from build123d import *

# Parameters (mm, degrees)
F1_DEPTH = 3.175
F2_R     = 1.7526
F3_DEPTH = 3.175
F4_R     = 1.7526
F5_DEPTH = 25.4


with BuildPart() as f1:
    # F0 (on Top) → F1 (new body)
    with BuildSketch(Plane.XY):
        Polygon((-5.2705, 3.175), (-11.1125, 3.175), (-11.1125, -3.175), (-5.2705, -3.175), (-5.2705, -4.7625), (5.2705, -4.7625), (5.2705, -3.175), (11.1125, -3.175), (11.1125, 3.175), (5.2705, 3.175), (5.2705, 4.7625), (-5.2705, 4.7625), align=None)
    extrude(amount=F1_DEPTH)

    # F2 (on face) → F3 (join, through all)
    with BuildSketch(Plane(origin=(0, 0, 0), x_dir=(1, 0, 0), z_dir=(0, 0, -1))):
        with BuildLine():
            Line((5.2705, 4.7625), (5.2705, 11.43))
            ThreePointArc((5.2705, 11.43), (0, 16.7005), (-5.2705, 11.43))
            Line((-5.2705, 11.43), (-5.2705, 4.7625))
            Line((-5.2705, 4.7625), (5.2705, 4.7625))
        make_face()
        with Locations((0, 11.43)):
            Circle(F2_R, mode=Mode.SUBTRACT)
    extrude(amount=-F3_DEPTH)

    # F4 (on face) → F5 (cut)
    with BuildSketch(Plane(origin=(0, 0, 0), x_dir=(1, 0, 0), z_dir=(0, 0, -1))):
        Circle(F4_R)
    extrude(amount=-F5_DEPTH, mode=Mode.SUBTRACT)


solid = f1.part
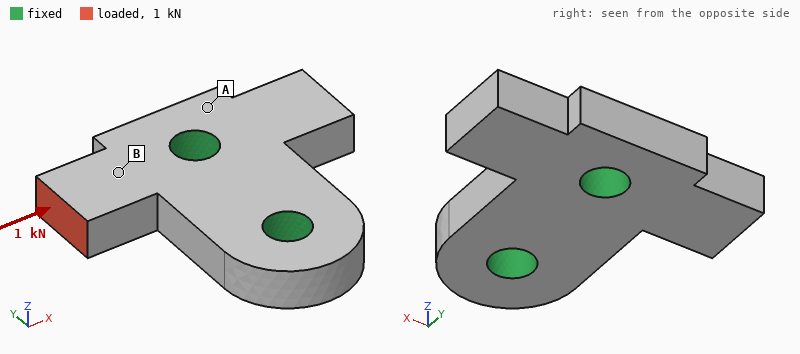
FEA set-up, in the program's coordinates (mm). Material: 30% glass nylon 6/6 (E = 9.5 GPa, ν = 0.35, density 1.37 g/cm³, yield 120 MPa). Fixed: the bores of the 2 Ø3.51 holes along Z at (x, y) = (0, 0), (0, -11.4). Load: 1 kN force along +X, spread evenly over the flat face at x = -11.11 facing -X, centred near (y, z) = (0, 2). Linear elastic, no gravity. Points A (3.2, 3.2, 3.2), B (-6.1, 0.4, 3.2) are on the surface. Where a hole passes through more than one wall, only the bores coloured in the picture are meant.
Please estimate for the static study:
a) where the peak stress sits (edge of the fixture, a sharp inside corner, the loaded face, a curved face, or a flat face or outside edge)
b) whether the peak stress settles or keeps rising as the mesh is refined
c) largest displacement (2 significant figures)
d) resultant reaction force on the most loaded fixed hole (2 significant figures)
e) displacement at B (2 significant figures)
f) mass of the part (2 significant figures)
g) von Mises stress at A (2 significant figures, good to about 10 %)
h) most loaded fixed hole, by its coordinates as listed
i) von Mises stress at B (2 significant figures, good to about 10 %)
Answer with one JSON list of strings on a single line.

["edge of the fixture", "keeps rising", "56 µm", "960 N", "26 µm", "1.2 g", "7.7 MPa", "(0, 0)", "46 MPa"]
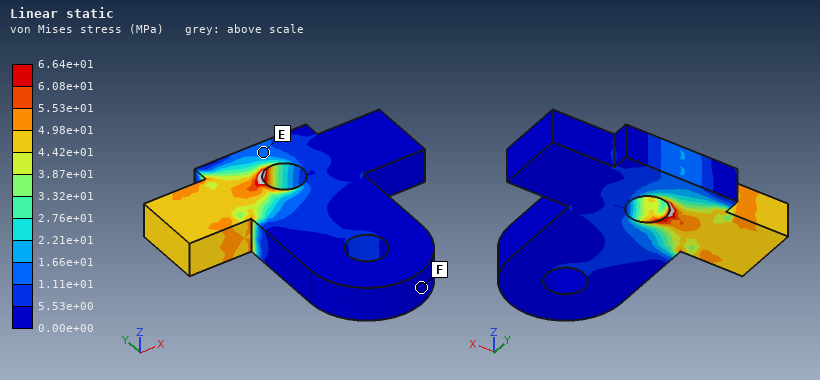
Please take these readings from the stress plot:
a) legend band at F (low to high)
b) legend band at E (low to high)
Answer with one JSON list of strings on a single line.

["0.00e+00 to 5.53e+00 MPa", "1.11e+01 to 1.66e+01 MPa"]
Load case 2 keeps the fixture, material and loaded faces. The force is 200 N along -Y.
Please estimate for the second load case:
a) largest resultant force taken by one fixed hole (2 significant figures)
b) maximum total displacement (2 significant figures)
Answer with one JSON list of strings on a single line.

["160 N", "98 µm"]
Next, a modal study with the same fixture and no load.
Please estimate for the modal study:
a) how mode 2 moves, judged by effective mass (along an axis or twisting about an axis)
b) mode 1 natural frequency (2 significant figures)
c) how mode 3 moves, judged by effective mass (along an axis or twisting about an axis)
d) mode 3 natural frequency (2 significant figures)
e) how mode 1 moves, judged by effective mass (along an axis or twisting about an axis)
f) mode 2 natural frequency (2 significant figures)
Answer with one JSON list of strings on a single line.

["along Z", "14 kHz", "twisting about Z", "25 kHz", "twisting about Y", "15 kHz"]
